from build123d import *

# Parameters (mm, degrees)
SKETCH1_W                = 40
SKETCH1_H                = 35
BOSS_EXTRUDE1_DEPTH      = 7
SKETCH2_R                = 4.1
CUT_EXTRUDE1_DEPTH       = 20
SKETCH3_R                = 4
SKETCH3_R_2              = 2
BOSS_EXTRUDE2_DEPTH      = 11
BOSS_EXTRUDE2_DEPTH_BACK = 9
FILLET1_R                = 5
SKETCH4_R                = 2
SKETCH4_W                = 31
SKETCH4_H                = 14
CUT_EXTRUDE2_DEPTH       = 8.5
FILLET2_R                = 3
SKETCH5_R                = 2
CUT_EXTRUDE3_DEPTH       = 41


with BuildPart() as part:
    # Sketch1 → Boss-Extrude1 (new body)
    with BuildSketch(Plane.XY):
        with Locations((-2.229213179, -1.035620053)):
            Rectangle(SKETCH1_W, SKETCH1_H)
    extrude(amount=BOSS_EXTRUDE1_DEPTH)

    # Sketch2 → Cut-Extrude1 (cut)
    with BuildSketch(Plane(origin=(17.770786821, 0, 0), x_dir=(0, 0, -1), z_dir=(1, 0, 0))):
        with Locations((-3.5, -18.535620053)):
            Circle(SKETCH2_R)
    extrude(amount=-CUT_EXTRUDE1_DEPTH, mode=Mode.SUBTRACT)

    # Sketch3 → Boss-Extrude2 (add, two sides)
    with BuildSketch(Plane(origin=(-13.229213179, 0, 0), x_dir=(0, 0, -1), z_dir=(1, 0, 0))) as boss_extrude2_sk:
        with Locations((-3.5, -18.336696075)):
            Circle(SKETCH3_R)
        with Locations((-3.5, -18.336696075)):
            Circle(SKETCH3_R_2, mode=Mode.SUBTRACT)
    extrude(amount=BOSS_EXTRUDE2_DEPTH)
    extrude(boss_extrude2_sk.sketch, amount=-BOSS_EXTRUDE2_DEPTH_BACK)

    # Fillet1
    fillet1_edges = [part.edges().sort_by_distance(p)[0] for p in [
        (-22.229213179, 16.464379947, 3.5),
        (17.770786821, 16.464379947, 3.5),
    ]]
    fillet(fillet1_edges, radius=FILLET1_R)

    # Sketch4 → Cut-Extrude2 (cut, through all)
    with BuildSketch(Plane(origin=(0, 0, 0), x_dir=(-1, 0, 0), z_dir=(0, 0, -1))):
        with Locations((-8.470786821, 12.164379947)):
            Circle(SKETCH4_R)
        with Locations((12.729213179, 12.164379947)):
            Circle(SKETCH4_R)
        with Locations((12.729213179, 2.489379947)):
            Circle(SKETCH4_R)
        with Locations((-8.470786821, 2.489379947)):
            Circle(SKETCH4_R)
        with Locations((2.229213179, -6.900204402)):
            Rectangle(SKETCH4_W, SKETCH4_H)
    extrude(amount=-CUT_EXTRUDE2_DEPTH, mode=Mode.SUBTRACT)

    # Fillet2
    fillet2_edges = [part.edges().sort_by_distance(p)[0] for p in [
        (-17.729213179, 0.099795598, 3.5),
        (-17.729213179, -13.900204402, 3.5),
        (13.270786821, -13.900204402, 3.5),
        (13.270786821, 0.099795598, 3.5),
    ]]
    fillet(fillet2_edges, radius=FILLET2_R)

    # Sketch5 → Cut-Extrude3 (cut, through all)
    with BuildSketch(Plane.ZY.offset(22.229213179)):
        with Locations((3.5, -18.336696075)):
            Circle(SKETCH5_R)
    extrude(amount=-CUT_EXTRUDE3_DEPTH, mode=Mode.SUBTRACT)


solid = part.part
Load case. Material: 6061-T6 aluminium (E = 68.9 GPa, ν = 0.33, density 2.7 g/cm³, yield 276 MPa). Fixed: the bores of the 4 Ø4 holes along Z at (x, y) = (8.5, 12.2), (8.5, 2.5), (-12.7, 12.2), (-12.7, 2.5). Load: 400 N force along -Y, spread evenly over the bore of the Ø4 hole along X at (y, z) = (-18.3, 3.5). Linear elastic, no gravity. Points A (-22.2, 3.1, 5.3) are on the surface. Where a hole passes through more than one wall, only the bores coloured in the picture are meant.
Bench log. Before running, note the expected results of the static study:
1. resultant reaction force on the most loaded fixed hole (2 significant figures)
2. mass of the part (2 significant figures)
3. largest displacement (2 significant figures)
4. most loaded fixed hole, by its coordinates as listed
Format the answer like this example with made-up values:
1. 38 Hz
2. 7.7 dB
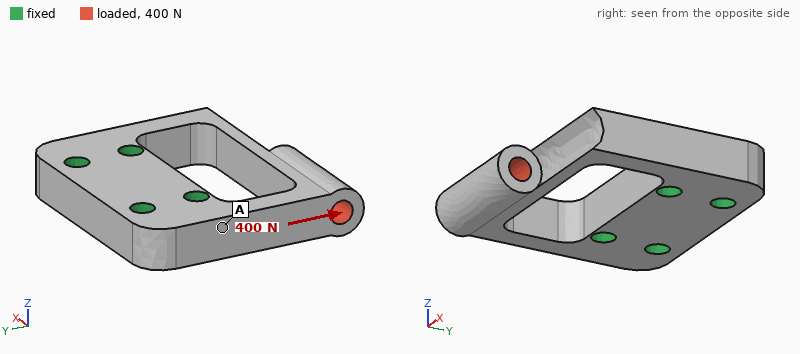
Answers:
1. 310 N
2. 17 g
3. 93 µm
4. (-12.7, 2.5)
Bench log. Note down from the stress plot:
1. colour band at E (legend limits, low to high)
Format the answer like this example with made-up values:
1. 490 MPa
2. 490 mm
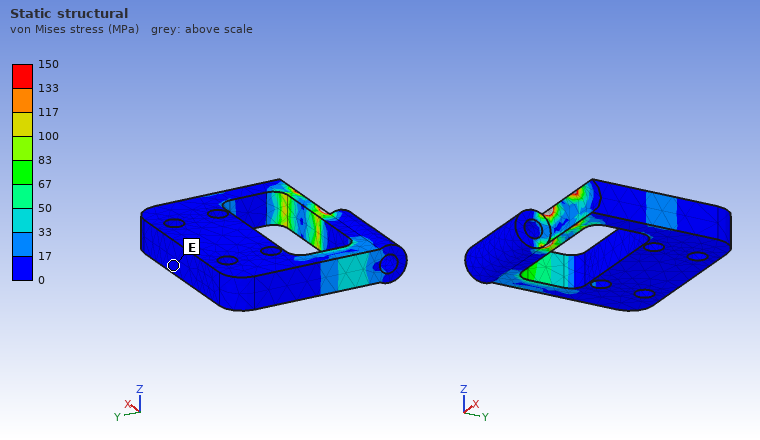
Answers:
1. 0 to 17 MPa
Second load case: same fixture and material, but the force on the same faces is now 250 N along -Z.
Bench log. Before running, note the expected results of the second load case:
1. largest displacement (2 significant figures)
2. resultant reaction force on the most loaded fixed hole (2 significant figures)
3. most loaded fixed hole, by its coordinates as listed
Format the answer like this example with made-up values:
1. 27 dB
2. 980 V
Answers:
1. 0.12 mm
2. 400 N
3. (-12.7, 2.5)
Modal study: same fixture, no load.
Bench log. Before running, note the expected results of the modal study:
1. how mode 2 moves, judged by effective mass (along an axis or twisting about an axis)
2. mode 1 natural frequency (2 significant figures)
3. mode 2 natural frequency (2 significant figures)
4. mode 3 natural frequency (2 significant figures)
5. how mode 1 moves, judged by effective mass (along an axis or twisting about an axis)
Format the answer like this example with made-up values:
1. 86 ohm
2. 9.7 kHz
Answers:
1. along X
2. 5100 Hz
3. 5800 Hz
4. 11 kHz
5. along Z
